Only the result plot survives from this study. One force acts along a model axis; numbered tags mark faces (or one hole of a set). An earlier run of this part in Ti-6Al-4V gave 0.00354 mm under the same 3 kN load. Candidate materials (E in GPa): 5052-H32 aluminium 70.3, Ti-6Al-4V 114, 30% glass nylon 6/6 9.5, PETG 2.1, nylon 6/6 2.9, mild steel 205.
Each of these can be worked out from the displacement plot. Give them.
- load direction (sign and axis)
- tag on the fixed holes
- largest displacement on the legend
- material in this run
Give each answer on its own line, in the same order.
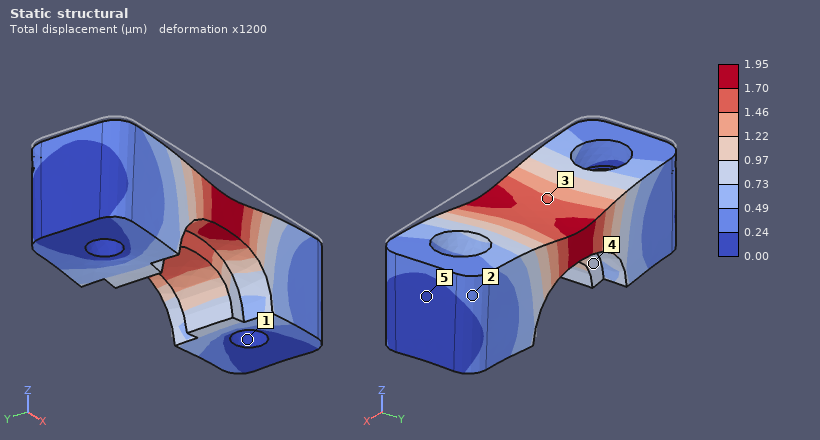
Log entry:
-Z
1
1.95 µm
mild steel
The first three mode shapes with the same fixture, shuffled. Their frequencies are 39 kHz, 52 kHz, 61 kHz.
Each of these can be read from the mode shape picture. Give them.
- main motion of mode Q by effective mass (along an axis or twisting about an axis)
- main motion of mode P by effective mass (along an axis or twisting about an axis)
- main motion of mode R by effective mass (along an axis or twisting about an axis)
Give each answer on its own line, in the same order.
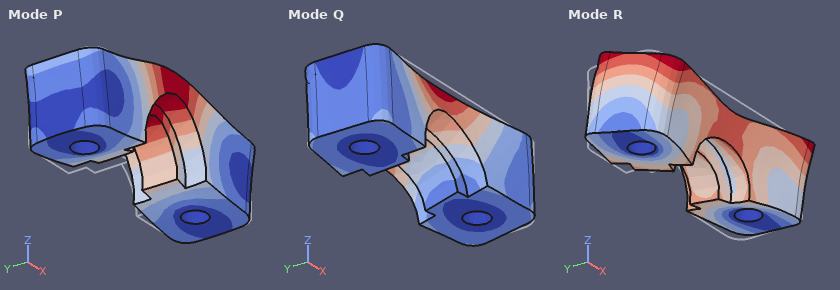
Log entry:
along Y
along Z
twisting about X
